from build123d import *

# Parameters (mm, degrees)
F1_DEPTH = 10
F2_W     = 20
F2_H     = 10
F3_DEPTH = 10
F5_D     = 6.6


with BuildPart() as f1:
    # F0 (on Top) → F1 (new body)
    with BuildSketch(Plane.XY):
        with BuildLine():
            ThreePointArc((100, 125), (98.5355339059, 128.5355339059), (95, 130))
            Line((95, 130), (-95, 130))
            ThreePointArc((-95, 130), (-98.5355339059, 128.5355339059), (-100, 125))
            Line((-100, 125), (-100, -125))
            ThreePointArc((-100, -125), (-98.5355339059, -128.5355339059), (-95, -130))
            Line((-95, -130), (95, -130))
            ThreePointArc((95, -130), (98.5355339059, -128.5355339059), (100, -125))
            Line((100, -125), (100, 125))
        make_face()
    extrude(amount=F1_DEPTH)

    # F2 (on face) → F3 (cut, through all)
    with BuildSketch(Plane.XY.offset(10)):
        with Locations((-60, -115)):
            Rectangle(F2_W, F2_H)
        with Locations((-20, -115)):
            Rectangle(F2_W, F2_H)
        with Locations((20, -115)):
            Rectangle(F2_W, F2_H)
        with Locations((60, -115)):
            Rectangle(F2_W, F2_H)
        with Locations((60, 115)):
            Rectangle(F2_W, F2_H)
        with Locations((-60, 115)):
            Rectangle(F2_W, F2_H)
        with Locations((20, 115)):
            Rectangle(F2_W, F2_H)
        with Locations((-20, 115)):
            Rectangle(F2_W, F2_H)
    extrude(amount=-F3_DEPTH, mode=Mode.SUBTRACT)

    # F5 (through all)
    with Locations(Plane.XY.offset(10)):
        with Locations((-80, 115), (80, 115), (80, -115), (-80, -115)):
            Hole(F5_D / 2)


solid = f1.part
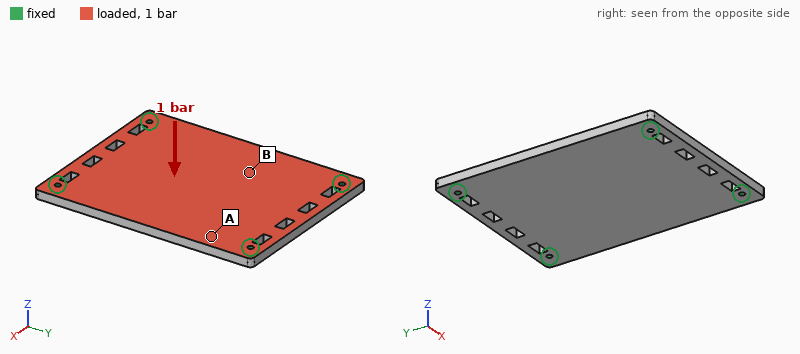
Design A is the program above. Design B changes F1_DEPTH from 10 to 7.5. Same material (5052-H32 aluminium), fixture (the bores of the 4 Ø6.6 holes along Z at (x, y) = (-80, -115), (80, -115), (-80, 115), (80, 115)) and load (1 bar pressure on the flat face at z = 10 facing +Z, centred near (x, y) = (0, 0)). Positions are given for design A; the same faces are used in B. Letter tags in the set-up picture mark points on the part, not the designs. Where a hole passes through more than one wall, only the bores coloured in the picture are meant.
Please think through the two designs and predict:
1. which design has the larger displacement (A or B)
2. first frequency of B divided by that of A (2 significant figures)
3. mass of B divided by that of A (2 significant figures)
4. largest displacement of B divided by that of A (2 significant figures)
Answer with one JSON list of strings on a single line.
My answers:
["B", "0.77", "0.75", "2.3"]
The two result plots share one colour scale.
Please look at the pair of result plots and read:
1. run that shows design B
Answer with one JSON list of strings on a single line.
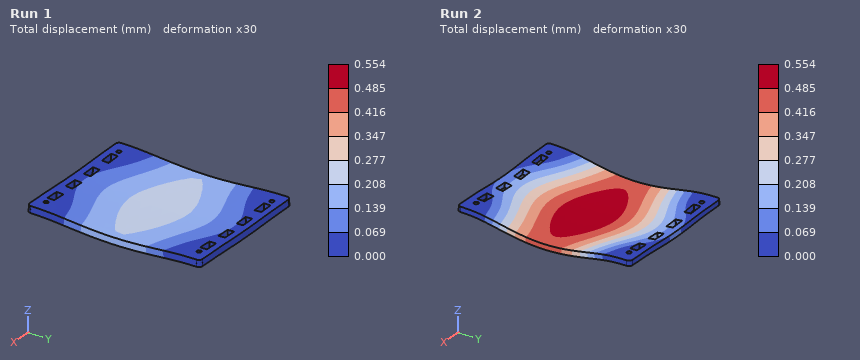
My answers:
["Run 2"]
